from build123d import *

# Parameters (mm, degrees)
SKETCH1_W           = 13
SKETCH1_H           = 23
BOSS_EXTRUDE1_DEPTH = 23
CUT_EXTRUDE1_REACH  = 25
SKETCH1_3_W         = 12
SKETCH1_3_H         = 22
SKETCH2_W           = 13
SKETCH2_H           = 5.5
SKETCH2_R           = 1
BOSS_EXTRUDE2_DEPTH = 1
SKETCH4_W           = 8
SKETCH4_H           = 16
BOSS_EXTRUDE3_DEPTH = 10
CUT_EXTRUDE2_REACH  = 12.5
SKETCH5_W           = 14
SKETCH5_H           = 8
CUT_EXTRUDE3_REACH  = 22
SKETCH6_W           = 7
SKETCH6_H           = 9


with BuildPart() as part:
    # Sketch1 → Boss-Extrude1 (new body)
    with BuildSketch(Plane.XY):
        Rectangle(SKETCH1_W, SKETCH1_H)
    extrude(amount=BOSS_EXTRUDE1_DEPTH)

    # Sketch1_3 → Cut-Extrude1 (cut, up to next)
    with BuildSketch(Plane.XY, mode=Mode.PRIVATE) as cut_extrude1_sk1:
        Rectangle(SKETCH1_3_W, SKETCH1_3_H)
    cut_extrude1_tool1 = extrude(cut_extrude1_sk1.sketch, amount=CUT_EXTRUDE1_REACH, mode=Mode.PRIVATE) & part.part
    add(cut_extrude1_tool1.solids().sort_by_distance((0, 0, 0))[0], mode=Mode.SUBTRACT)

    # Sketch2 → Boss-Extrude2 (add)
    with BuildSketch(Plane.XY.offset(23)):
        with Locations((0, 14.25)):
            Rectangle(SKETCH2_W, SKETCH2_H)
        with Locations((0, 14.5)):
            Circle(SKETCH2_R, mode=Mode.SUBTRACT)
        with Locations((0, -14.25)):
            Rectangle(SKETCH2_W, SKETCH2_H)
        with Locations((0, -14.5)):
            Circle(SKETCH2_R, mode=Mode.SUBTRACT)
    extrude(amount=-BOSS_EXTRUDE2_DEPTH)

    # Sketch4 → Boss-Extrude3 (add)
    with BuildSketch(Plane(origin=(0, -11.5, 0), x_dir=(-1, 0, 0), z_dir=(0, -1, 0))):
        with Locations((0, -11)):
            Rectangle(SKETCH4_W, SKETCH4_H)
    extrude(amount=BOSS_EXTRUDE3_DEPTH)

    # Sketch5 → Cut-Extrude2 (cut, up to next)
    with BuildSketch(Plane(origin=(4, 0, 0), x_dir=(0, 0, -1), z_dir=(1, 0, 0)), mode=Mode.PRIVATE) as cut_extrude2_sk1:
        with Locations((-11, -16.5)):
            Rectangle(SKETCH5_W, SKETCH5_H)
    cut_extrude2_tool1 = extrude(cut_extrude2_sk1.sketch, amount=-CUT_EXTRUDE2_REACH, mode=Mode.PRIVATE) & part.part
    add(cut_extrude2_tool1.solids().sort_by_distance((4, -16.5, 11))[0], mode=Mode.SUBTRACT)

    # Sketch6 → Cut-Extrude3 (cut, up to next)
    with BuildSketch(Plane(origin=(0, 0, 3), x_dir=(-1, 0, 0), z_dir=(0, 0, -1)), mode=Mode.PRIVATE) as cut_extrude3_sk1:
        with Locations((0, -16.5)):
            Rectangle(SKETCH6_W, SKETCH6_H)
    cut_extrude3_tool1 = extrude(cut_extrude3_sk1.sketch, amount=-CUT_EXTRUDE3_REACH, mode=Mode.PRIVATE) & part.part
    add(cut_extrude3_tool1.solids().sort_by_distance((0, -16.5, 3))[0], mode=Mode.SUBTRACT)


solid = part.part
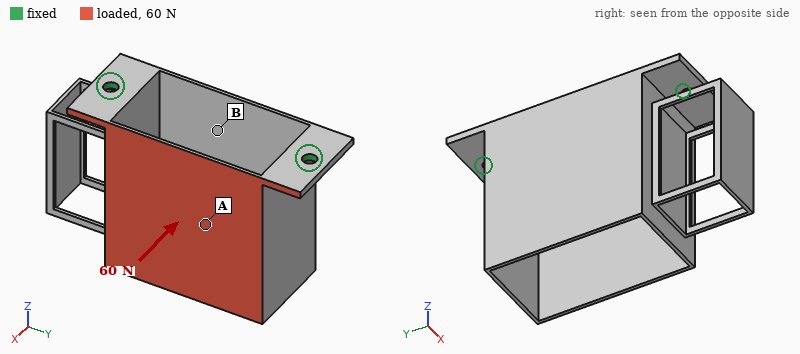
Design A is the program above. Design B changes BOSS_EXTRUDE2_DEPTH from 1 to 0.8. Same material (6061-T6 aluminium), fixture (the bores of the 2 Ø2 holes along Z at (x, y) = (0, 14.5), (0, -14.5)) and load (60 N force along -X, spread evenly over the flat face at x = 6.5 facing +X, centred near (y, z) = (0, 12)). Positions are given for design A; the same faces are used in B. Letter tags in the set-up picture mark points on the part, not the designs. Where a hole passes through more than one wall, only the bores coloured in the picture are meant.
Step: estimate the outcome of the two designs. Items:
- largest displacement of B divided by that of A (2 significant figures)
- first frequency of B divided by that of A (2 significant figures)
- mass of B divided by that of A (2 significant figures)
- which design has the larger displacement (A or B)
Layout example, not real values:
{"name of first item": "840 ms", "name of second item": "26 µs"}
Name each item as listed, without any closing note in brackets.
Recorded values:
{"largest displacement of B divided by that of A": "1.4", "first frequency of B divided by that of A": "0.80", "mass of B divided by that of A": "0.98", "which design has the larger displacement": "B"}
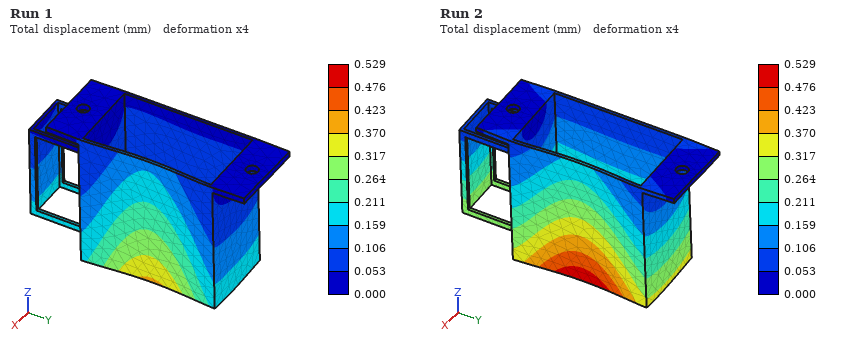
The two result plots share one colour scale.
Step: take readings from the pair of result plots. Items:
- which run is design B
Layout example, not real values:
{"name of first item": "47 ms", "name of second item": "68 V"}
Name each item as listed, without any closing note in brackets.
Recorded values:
{"which run is design B": "Run 2"}
